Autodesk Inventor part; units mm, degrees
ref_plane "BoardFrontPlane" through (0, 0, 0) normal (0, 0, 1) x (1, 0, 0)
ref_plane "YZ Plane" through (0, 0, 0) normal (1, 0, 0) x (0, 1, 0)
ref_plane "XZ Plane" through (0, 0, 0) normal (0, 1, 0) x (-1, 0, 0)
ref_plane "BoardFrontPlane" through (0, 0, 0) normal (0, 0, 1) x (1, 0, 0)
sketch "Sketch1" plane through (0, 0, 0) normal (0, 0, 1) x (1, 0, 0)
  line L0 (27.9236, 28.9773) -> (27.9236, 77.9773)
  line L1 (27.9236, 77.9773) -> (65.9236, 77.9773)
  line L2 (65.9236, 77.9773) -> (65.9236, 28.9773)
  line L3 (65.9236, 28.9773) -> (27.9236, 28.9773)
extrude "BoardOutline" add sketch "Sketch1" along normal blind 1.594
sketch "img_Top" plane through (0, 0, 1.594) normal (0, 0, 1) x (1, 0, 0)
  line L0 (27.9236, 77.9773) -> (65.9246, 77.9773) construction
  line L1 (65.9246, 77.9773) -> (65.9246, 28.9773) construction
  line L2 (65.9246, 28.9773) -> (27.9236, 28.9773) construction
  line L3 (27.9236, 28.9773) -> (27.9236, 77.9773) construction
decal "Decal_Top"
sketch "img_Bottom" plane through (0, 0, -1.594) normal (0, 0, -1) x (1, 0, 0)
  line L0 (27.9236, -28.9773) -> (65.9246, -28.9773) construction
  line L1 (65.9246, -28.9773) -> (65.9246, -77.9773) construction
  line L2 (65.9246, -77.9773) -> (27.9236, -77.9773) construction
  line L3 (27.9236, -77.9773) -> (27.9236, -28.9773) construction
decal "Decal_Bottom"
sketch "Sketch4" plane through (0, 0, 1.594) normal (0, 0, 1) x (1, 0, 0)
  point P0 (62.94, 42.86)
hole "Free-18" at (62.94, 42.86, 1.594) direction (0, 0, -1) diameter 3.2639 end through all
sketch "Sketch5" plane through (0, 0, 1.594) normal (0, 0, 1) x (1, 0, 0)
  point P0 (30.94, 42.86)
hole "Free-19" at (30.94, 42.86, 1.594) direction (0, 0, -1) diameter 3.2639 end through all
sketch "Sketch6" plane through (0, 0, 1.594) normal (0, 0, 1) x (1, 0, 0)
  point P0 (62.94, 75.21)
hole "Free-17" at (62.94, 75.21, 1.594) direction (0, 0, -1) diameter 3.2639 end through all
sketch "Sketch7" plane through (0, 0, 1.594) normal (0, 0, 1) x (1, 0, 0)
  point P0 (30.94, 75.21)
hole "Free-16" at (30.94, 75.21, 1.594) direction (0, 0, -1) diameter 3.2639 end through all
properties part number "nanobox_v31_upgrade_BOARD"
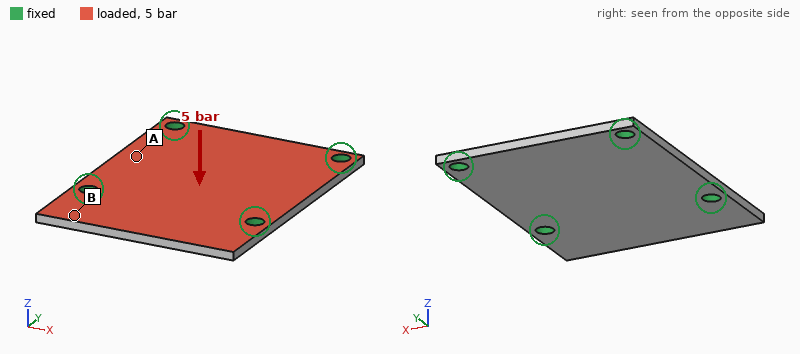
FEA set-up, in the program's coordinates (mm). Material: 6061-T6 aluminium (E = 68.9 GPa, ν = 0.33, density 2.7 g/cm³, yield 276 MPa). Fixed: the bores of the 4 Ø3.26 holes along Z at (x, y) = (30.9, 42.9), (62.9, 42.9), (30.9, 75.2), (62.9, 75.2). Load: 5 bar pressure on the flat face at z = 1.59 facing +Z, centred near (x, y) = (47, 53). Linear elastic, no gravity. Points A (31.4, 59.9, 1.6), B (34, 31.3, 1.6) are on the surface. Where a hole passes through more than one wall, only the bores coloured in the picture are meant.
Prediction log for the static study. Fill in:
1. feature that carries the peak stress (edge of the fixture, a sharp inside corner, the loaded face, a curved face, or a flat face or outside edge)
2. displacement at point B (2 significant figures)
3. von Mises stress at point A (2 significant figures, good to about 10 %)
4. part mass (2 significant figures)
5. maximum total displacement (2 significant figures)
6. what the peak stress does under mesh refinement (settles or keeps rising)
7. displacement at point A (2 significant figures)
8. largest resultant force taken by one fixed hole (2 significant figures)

edge of the fixture
0.086 mm
53 MPa
7.9 g
0.16 mm
keeps rising
0.063 mm
290 N
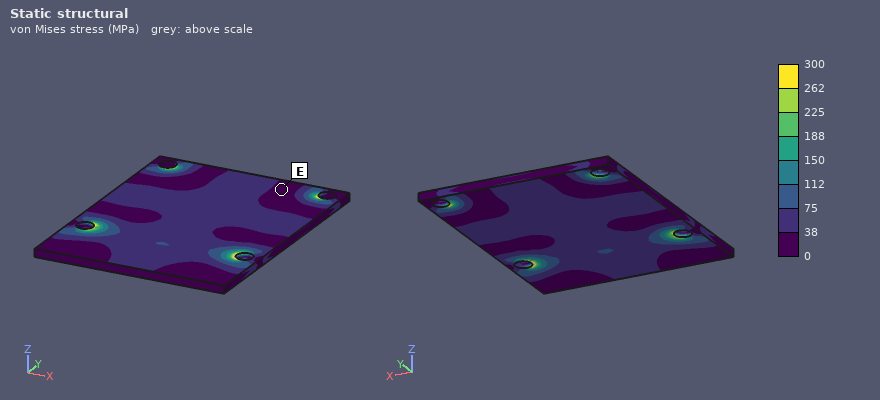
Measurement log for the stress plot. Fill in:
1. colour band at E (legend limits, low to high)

0 to 38 MPa
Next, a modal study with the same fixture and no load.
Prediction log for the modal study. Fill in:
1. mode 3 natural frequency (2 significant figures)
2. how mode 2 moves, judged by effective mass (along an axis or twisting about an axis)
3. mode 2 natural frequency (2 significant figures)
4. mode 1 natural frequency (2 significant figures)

9400 Hz
along Z
6000 Hz
5200 Hz
